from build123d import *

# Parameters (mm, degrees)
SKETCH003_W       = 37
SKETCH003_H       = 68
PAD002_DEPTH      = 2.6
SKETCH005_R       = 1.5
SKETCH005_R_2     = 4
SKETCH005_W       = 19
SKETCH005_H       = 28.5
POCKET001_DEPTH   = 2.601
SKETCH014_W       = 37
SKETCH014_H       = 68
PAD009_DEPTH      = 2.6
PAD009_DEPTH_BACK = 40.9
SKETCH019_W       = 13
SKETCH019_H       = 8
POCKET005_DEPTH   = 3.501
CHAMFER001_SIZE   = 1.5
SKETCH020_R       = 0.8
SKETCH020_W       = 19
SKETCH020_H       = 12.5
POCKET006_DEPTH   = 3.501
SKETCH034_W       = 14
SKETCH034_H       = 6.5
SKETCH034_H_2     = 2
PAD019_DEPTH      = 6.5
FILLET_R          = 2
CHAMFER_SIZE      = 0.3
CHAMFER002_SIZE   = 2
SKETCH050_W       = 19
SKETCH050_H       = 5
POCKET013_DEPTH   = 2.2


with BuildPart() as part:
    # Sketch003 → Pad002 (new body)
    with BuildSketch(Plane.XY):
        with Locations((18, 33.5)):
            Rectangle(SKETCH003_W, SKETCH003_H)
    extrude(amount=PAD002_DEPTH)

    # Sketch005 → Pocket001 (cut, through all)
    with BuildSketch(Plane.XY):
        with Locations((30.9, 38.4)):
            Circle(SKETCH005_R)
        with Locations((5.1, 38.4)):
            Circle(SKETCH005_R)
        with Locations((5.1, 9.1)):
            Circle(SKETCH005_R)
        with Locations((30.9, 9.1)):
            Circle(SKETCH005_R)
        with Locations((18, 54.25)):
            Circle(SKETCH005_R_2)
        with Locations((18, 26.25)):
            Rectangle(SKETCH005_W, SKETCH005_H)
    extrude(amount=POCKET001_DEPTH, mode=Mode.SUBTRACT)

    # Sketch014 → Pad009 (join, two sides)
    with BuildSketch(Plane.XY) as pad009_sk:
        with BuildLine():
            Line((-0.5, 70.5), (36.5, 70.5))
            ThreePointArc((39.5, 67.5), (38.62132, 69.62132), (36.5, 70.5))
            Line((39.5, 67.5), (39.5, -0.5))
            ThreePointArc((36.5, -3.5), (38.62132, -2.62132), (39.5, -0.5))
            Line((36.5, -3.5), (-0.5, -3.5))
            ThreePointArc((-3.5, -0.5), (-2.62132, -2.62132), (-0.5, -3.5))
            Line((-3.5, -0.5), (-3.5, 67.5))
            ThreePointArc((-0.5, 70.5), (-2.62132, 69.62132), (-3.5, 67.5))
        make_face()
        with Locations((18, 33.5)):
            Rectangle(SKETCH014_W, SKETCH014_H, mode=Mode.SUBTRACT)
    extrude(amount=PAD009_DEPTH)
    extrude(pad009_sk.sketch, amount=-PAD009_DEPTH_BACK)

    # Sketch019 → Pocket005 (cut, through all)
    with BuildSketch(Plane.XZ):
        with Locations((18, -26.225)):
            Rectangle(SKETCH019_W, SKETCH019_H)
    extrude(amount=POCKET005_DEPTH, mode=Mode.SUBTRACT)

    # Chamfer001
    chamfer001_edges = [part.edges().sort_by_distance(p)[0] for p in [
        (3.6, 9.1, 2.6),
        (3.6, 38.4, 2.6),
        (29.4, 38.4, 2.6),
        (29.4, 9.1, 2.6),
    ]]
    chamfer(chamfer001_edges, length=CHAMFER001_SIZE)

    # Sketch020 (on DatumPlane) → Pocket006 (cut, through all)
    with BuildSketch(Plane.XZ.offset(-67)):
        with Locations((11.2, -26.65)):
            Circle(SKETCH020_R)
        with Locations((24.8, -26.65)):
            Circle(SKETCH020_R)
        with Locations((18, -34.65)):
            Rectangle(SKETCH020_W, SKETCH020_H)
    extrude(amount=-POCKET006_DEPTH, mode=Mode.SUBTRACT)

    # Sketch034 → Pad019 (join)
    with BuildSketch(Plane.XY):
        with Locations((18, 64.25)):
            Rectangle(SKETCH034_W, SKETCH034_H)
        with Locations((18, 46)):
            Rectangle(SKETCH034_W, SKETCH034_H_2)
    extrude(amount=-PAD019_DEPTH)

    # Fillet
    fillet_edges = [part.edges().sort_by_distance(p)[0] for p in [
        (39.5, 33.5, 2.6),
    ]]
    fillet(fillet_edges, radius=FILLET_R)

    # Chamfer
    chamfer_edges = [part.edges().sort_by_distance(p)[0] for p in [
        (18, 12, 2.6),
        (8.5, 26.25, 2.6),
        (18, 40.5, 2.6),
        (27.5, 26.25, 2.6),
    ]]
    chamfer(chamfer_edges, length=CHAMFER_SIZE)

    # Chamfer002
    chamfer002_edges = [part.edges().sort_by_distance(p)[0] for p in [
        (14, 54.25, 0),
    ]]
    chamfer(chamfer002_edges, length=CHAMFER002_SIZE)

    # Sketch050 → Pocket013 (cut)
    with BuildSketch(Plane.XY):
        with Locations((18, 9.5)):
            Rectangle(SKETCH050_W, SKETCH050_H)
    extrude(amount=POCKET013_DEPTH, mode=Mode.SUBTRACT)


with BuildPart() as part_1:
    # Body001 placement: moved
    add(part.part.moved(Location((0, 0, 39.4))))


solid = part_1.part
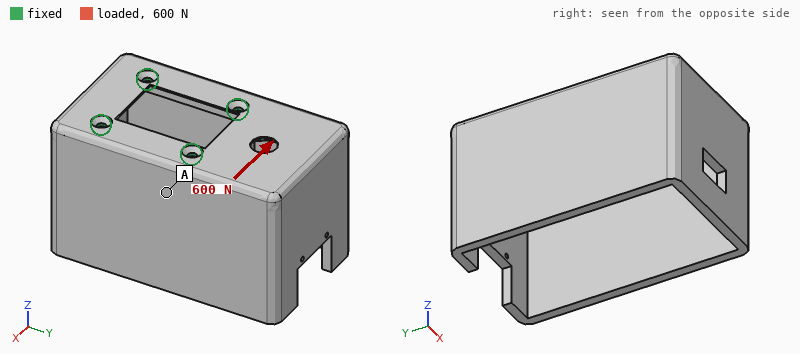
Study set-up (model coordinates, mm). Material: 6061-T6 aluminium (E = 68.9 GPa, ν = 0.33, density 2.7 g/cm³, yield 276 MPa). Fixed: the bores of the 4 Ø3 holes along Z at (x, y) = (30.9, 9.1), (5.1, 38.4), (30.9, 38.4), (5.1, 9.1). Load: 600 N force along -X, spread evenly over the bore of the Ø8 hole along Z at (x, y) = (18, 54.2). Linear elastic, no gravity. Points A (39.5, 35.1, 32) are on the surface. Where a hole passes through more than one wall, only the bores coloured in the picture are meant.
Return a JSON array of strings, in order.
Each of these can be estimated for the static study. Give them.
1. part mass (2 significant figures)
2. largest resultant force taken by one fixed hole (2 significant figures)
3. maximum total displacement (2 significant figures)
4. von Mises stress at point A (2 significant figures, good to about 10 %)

["89 g", "370 N", "10 µm", "3.9 MPa"]
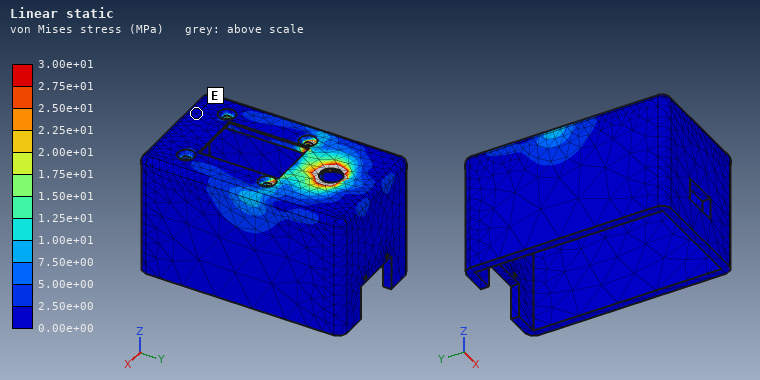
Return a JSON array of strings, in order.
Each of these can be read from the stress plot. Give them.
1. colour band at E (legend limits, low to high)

["0.00e+00 to 2.50e+00 MPa"]
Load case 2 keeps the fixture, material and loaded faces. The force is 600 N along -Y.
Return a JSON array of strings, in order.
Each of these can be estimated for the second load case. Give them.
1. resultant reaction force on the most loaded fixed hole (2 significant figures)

["270 N"]
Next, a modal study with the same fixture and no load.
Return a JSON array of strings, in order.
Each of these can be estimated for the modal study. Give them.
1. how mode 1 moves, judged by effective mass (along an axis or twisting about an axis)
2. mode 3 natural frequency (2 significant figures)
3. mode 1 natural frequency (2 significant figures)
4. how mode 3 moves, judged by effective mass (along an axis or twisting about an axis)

["along X", "2300 Hz", "1700 Hz", "along X"]
